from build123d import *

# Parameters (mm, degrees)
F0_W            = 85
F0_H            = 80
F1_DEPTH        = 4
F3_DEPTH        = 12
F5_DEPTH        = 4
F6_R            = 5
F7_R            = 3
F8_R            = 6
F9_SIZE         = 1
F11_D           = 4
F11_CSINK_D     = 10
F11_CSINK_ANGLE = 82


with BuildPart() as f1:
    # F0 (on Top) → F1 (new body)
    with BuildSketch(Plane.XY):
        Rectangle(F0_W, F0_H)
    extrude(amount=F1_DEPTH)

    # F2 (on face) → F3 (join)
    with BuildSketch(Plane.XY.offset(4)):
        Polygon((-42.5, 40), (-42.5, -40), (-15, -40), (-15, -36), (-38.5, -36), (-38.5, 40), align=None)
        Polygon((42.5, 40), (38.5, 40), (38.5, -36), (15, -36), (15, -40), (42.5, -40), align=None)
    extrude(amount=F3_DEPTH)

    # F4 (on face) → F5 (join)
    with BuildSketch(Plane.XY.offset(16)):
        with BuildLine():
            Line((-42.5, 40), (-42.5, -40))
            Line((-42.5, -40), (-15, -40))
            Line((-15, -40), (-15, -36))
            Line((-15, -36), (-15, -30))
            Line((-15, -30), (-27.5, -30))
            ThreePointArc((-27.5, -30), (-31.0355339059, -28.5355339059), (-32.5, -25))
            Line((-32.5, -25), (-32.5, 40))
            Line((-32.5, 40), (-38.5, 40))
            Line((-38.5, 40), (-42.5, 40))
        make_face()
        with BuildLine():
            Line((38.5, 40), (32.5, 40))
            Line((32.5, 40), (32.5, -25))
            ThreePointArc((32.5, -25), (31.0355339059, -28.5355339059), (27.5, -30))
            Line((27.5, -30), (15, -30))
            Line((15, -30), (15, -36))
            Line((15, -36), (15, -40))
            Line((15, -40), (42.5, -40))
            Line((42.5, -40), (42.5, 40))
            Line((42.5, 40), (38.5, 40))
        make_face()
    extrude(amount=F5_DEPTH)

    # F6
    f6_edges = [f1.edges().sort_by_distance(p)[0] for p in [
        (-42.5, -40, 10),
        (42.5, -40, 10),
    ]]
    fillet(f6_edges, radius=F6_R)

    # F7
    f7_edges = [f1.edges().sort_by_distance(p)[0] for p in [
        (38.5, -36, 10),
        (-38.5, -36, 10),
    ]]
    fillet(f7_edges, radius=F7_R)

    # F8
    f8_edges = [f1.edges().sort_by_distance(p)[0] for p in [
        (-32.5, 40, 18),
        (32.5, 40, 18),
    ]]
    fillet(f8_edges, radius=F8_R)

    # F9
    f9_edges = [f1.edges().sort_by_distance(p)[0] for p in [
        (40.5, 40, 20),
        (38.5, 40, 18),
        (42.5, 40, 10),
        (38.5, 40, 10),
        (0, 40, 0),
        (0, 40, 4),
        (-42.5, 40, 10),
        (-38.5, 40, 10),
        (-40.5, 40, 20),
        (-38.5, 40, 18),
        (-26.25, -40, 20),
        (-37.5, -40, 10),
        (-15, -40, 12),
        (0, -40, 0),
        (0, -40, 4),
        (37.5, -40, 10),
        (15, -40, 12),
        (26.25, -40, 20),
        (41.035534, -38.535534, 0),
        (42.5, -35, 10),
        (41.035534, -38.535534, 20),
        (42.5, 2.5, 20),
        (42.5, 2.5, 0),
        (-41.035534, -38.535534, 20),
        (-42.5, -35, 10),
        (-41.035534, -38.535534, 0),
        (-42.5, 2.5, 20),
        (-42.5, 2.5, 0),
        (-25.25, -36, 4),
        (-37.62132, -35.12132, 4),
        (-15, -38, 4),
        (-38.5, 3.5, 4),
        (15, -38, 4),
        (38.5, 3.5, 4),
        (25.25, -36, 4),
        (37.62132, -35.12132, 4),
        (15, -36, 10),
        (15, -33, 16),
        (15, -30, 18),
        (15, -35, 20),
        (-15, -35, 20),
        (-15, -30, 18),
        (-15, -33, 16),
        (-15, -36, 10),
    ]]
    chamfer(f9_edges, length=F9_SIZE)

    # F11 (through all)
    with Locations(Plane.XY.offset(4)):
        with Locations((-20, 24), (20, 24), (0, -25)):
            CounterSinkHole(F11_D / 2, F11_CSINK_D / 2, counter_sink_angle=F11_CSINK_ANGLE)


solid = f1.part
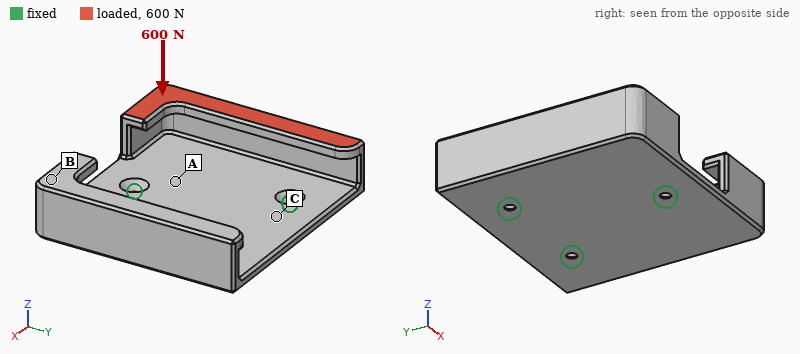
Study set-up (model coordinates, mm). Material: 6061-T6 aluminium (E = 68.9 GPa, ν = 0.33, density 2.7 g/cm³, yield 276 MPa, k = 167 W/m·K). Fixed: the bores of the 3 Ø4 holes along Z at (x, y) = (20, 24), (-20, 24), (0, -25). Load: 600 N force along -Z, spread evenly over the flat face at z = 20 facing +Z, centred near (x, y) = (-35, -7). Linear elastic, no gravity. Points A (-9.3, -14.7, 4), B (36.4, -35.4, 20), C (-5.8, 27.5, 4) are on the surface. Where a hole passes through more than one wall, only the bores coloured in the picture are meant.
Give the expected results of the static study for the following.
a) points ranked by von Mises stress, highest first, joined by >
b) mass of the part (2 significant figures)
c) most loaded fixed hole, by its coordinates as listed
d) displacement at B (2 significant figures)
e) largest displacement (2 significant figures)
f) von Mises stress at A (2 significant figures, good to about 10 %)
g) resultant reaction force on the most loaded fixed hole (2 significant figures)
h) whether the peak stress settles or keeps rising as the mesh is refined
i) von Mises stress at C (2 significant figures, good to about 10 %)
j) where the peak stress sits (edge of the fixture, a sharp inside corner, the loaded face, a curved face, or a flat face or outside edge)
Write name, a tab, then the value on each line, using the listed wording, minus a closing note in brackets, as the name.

points ranked by von Mises stress, highest first, joined by >	A > C > B
mass of the part	120 g
most loaded fixed hole, by its coordinates as listed	(20, 24)
displacement at B	0.13 mm
largest displacement	0.54 mm
von Mises stress at A	56 MPa
resultant reaction force on the most loaded fixed hole	1.1 kN
whether the peak stress settles or keeps rising as the mesh is refined	keeps rising
von Mises stress at C	29 MPa
where the peak stress sits	edge of the fixture
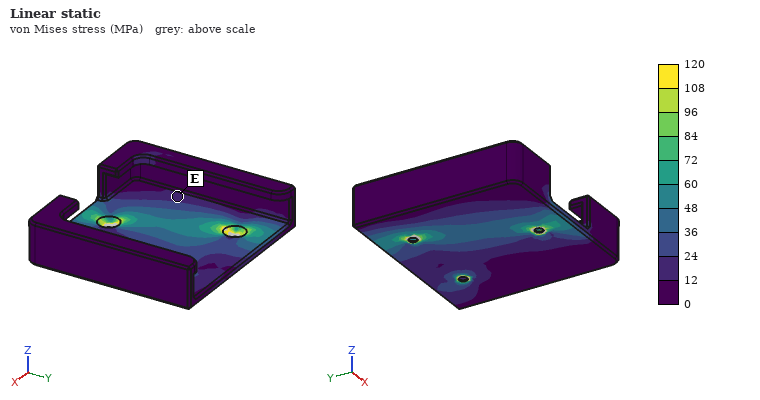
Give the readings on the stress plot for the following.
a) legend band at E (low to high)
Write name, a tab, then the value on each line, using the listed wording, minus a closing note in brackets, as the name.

legend band at E	12 to 24 MPa
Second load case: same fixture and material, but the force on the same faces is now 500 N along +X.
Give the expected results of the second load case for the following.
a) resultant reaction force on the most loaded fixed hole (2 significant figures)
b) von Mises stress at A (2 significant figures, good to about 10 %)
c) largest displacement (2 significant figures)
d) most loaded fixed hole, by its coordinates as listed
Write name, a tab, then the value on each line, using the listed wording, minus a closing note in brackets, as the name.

resultant reaction force on the most loaded fixed hole	750 N
von Mises stress at A	34 MPa
largest displacement	0.37 mm
most loaded fixed hole, by its coordinates as listed	(20, 24)
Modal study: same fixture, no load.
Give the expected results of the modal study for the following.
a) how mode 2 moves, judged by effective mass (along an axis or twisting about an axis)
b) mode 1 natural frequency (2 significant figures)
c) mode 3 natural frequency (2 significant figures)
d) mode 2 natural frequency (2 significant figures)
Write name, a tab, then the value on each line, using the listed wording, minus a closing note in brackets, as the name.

how mode 2 moves, judged by effective mass	along Z
mode 1 natural frequency	900 Hz
mode 3 natural frequency	2400 Hz
mode 2 natural frequency	1200 Hz
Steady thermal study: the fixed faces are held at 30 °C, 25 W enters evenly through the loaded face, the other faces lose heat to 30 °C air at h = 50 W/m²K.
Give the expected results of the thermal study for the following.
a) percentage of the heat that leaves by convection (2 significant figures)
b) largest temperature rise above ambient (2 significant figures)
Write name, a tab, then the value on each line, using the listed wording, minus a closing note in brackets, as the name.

percentage of the heat that leaves by convection	34 %
largest temperature rise above ambient	21 K
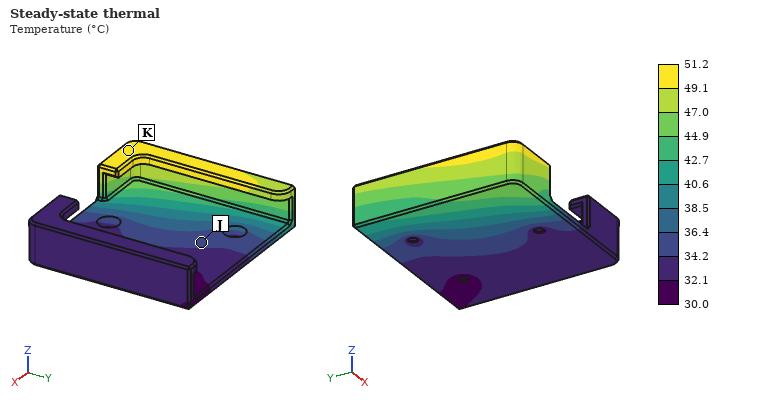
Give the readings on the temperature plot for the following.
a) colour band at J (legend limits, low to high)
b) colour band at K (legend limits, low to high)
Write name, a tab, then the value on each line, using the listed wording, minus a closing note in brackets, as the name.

colour band at J	34.2 to 36.4 °C
colour band at K	49.1 to 51.2 °C
